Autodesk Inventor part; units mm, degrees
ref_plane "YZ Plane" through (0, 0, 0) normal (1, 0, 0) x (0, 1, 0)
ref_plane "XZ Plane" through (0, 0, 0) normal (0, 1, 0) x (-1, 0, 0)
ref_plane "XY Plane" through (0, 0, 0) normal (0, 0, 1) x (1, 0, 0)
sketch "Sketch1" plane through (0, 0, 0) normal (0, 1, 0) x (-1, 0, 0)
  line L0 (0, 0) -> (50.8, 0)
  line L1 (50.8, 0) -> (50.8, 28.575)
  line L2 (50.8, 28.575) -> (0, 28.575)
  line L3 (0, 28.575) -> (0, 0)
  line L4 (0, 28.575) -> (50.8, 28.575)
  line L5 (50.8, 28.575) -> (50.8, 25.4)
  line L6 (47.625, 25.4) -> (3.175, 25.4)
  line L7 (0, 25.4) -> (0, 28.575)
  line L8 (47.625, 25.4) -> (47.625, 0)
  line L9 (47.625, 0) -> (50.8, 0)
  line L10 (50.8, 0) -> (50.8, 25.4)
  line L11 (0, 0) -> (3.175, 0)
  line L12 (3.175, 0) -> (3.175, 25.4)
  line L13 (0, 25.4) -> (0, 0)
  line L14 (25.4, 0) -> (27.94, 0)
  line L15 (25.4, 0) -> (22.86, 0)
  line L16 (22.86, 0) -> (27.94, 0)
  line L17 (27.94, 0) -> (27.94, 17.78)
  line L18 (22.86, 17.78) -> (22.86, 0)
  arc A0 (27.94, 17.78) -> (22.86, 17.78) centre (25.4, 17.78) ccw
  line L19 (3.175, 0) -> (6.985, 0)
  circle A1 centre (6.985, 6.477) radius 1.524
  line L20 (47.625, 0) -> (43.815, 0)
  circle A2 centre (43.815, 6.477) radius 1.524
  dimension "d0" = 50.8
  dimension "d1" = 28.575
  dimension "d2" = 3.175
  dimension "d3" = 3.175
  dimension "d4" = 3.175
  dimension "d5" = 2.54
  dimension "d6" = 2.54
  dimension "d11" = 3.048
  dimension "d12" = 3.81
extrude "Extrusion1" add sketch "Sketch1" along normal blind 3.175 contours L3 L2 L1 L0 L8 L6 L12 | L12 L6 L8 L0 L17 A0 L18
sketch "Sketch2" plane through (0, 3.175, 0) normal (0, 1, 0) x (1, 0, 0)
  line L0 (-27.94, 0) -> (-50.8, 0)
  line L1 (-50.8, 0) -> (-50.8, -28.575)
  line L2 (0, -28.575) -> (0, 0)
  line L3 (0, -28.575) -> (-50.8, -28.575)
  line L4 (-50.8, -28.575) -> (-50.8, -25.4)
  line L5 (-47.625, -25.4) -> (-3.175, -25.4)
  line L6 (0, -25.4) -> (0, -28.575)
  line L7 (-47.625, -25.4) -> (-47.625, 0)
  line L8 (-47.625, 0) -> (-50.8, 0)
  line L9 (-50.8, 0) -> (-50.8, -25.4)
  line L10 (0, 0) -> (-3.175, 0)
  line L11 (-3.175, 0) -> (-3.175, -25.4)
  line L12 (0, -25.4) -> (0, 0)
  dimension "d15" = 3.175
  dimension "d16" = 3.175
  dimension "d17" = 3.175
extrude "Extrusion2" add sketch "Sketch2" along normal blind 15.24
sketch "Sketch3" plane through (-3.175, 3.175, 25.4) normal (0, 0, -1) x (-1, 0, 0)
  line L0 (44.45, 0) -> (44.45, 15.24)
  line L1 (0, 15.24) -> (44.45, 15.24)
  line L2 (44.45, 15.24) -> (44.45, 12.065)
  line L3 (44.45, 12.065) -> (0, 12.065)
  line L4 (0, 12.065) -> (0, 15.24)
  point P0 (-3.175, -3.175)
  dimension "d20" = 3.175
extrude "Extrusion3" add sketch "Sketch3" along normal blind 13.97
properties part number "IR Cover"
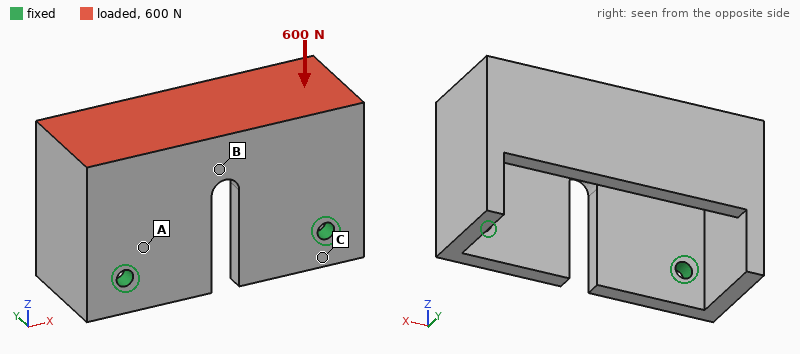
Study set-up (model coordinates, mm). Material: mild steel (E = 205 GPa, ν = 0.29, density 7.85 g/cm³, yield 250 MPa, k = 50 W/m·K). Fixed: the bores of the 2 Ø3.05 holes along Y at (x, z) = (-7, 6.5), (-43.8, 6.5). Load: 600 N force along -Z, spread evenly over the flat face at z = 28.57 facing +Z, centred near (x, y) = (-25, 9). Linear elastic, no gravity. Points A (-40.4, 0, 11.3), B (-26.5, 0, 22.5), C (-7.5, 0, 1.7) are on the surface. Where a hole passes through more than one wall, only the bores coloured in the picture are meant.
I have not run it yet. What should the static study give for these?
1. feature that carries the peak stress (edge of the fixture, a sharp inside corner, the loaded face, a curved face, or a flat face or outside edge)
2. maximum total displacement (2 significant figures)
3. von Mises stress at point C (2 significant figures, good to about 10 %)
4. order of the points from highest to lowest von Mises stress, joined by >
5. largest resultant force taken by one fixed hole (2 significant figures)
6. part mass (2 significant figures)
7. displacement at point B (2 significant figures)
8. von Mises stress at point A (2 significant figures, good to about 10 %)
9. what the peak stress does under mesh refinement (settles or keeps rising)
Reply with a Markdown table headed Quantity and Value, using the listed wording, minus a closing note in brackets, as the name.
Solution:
| Quantity | Value |
|---|---|
| feature that carries the peak stress | edge of the fixture |
| maximum total displacement | 21 µm |
| von Mises stress at point C | 31 MPa |
| order of the points from highest to lowest von Mises stress, joined by > | C > A > B |
| largest resultant force taken by one fixed hole | 300 N |
| part mass | 87 g |
| displacement at point B | 10 µm |
| von Mises stress at point A | 19 MPa |
| what the peak stress does under mesh refinement | keeps rising |
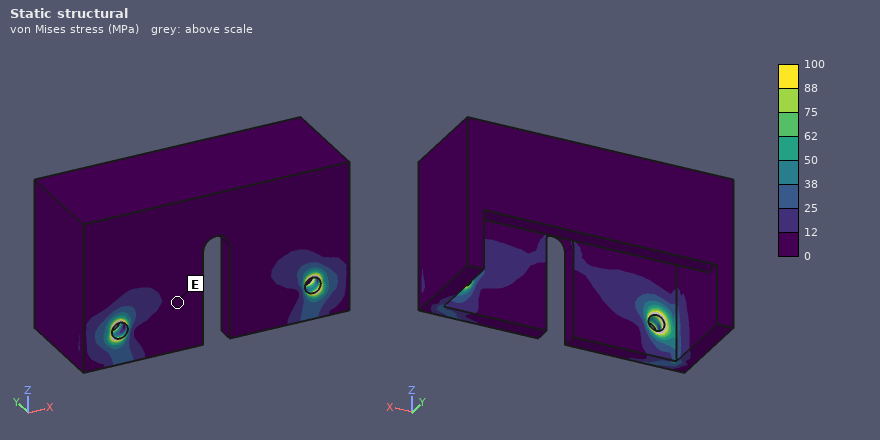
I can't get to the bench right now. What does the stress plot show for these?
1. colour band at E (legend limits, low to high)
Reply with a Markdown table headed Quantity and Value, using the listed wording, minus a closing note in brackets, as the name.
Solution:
| Quantity | Value |
|---|---|
| colour band at E | 0 to 12 MPa |
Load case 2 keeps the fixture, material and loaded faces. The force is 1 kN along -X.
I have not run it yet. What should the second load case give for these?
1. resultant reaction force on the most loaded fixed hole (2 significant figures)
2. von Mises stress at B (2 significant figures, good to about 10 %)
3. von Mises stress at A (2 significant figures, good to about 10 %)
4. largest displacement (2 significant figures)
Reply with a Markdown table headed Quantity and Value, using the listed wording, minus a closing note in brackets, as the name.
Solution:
| Quantity | Value |
|---|---|
| resultant reaction force on the most loaded fixed hole | 750 N |
| von Mises stress at B | 25 MPa |
| von Mises stress at A | 21 MPa |
| largest displacement | 15 µm |
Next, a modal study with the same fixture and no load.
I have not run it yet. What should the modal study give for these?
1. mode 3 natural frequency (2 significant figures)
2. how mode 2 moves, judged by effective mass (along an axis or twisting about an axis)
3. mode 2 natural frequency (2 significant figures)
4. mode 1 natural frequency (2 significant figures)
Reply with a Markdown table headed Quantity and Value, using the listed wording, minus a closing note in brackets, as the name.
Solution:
| Quantity | Value |
|---|---|
| mode 3 natural frequency | 9600 Hz |
| how mode 2 moves, judged by effective mass | along X |
| mode 2 natural frequency | 4000 Hz |
| mode 1 natural frequency | 2600 Hz |
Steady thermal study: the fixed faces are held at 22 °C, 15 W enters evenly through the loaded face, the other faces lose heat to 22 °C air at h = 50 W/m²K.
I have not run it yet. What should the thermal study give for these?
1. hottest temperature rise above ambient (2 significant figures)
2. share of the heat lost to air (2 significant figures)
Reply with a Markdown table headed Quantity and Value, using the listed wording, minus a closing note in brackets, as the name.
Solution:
| Quantity | Value |
|---|---|
| hottest temperature rise above ambient | 29 K |
| share of the heat lost to air | 37 % |
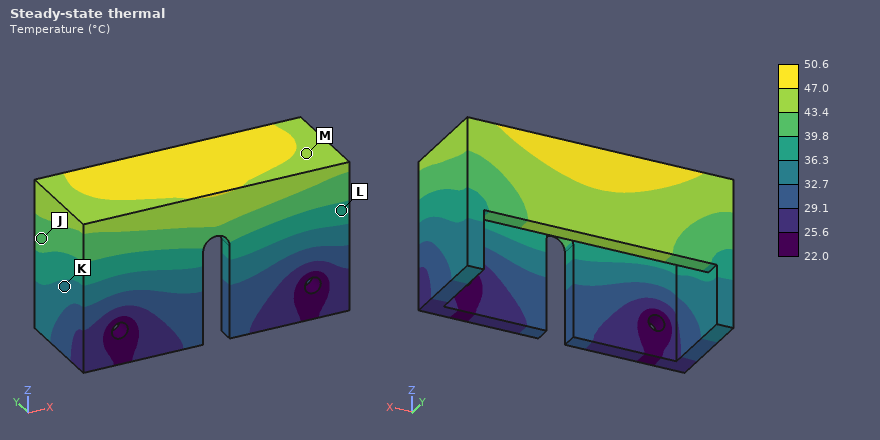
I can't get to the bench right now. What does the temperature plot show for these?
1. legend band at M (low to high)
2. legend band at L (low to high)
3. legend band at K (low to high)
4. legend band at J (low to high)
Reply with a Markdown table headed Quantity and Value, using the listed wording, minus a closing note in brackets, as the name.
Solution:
| Quantity | Value |
|---|---|
| legend band at M | 43.4 to 47.0 °C |
| legend band at L | 36.3 to 39.8 °C |
| legend band at K | 32.7 to 36.3 °C |
| legend band at J | 39.8 to 43.4 °C |
